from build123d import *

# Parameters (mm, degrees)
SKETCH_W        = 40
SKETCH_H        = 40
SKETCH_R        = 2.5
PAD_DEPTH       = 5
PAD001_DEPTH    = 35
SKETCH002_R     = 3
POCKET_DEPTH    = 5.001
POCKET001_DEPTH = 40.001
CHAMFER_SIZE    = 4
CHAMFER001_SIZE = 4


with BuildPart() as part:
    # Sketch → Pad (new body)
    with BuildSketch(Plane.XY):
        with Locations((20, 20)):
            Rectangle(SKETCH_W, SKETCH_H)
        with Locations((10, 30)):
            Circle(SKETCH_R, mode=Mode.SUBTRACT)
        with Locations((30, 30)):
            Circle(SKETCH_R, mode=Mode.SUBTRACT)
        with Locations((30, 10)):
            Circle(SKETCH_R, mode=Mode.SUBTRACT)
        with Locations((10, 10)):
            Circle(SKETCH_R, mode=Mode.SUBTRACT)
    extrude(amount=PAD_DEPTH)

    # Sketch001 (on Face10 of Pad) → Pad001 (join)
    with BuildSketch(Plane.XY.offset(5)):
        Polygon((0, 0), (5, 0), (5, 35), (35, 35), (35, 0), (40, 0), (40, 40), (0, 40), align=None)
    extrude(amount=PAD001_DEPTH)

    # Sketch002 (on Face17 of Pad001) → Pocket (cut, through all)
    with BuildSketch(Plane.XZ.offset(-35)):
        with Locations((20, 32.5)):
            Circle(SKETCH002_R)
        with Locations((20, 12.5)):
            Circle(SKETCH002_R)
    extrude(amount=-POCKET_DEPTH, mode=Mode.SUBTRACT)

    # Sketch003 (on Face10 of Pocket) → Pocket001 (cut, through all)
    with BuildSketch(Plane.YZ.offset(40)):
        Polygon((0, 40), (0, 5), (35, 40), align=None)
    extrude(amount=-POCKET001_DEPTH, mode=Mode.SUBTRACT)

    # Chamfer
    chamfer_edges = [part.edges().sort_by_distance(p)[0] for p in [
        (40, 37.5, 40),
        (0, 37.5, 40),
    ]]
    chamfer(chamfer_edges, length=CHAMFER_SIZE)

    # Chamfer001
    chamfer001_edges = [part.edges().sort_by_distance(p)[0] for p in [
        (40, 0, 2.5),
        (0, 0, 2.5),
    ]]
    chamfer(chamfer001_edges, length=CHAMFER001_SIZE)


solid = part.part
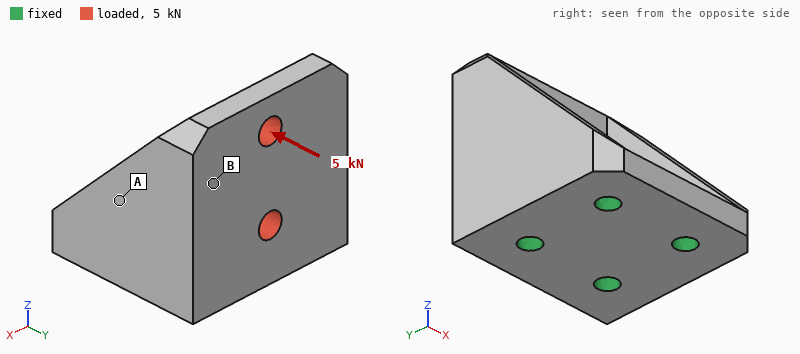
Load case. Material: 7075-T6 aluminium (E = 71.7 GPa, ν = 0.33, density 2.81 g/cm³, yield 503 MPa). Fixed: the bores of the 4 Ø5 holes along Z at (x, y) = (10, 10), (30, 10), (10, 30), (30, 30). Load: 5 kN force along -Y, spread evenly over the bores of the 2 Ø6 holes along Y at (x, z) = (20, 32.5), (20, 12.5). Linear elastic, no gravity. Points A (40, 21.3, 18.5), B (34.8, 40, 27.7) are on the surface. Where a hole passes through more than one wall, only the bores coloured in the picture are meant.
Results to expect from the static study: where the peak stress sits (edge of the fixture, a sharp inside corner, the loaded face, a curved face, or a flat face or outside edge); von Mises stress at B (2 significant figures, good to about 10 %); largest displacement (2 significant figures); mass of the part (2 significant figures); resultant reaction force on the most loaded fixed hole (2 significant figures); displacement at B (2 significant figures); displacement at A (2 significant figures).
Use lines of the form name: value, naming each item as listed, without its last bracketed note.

where the peak stress sits: the loaded face
von Mises stress at B: 57 MPa
largest displacement: 0.22 mm
mass of the part: 57 g
resultant reaction force on the most loaded fixed hole: 2.5 kN
displacement at B: 0.078 mm
displacement at A: 0.052 mm
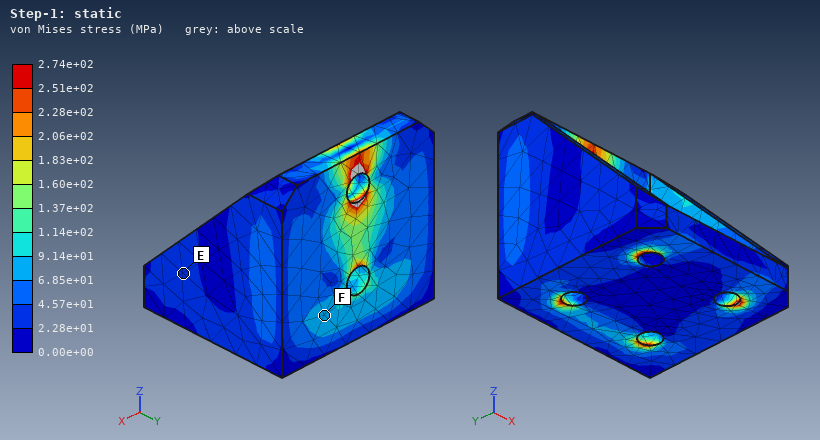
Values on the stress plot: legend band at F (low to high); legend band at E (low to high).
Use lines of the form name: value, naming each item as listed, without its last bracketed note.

legend band at F: 6.85e+01 to 9.14e+01 MPa
legend band at E: 2.28e+01 to 4.57e+01 MPa
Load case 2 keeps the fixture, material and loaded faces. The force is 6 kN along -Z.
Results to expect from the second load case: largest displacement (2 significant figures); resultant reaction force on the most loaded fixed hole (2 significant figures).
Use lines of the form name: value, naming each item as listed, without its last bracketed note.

largest displacement: 54 µm
resultant reaction force on the most loaded fixed hole: 3.5 kN
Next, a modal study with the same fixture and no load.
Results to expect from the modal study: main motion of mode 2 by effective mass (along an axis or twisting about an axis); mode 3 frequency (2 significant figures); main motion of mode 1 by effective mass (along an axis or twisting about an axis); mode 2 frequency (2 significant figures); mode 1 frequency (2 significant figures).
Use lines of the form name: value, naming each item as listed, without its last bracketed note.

main motion of mode 2 by effective mass: along Y
mode 3 frequency: 13 kHz
main motion of mode 1 by effective mass: along X
mode 2 frequency: 7700 Hz
mode 1 frequency: 6800 Hz
